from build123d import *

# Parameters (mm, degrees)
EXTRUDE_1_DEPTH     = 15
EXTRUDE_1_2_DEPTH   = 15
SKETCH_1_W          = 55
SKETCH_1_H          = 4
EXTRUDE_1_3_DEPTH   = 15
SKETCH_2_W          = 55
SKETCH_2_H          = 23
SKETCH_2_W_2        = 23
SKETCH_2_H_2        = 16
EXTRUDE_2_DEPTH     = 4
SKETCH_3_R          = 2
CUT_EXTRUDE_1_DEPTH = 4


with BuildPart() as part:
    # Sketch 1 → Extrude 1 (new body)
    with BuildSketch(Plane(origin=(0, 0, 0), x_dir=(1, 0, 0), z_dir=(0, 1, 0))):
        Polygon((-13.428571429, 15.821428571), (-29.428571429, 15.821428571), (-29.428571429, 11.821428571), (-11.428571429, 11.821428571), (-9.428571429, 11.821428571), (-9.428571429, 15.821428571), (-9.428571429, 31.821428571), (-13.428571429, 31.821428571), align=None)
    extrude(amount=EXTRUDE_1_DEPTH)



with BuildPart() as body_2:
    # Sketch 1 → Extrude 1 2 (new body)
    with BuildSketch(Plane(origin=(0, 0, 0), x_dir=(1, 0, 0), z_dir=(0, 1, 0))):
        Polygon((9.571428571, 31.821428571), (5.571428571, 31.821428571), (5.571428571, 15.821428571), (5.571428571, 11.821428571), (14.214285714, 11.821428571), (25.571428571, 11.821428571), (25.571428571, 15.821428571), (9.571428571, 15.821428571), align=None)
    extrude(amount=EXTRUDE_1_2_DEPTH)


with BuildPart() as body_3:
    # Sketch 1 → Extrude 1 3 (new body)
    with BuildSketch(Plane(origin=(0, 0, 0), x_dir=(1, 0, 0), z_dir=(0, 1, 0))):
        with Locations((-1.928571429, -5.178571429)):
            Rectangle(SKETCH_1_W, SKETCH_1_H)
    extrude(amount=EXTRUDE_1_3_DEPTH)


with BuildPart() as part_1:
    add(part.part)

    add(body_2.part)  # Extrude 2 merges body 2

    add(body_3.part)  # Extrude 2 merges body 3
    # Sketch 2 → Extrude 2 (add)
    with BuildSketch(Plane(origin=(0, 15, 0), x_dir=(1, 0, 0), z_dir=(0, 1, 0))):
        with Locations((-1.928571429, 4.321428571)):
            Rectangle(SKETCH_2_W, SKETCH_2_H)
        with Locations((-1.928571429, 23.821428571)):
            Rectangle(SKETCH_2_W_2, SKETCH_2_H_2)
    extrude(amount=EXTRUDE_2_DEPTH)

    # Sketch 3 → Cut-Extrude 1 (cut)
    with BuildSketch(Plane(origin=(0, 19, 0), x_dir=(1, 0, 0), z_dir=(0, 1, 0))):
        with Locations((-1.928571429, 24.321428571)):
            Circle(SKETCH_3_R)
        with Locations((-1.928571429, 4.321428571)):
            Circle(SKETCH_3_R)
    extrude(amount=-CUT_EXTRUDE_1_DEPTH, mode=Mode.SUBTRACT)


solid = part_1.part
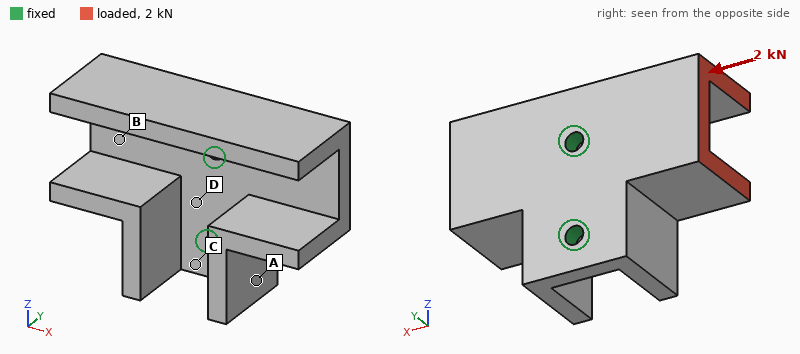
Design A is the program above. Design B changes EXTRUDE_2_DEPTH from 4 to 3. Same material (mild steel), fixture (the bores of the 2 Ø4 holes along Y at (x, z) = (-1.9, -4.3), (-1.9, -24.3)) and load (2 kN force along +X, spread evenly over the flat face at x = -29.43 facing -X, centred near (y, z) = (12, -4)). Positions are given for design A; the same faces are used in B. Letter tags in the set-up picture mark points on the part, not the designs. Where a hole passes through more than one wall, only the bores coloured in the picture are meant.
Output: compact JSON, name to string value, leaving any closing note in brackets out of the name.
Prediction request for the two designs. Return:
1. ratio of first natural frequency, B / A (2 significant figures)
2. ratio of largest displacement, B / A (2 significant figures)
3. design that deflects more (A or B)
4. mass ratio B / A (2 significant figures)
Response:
{"ratio of first natural frequency, B / A": "0.75", "ratio of largest displacement, B / A": "2.0", "design that deflects more": "B", "mass ratio B / A": "0.89"}
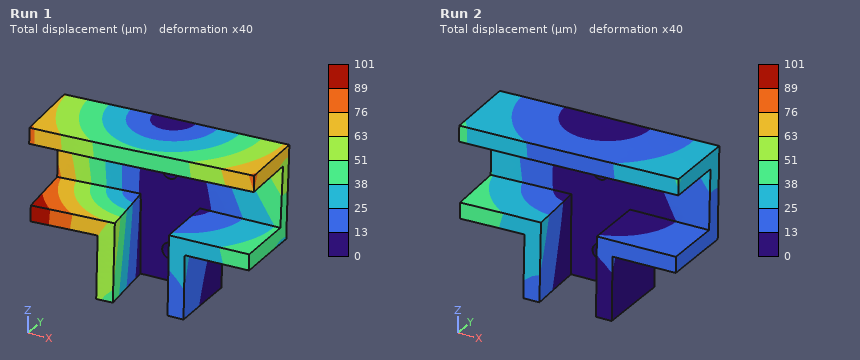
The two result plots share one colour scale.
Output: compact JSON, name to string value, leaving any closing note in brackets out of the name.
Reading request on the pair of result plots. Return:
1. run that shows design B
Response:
{"run that shows design B": "Run 1"}
